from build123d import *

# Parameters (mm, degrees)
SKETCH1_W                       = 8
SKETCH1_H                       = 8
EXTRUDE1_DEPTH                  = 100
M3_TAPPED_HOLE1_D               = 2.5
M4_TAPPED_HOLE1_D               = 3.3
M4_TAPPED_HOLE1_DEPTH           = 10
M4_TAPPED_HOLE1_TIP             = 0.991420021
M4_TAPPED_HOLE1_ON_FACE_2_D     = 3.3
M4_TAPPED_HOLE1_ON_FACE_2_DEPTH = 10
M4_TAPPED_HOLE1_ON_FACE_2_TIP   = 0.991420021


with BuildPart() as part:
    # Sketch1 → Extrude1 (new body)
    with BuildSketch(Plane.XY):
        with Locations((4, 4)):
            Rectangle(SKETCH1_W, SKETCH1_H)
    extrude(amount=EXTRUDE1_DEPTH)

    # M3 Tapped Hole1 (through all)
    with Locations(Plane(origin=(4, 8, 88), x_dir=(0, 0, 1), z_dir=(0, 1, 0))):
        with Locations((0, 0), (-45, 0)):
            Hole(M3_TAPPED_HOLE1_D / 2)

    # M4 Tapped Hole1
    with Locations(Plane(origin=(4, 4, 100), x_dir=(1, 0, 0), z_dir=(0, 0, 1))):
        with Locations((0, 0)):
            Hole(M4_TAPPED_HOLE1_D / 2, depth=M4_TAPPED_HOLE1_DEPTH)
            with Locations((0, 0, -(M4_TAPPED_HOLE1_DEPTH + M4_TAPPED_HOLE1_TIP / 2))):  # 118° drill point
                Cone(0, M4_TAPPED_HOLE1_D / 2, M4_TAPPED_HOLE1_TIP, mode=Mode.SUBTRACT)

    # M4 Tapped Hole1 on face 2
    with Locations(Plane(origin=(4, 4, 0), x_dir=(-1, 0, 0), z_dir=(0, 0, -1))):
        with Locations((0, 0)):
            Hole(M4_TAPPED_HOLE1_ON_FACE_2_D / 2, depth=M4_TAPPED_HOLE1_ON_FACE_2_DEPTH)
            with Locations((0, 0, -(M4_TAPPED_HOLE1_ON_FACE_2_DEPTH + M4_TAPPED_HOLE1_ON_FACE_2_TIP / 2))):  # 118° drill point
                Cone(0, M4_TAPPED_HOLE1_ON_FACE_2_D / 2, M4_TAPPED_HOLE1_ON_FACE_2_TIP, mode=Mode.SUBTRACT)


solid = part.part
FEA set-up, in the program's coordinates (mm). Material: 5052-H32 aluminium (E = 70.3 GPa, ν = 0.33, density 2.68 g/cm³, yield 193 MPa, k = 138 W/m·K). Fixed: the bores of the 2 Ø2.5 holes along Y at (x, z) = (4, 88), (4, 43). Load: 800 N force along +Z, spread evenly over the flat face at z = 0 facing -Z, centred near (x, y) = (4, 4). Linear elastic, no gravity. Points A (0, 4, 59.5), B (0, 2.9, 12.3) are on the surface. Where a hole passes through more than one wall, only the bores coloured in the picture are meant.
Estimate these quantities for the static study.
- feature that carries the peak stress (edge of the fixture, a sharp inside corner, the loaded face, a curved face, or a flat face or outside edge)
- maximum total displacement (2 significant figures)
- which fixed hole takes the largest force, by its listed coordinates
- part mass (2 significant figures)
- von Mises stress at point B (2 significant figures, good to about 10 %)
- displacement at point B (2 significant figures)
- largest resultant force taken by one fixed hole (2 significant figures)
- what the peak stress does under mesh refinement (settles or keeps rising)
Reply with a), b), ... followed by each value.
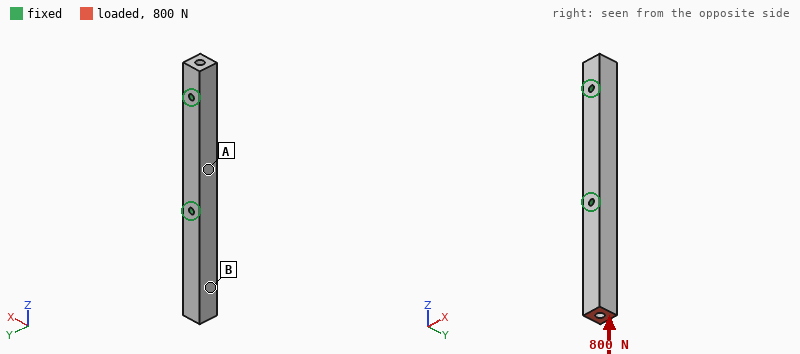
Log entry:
a) edge of the fixture
b) 8.1 µm
c) (4, 43)
d) 16 g
e) 13 MPa
f) 5.6 µm
g) 780 N
h) keeps rising
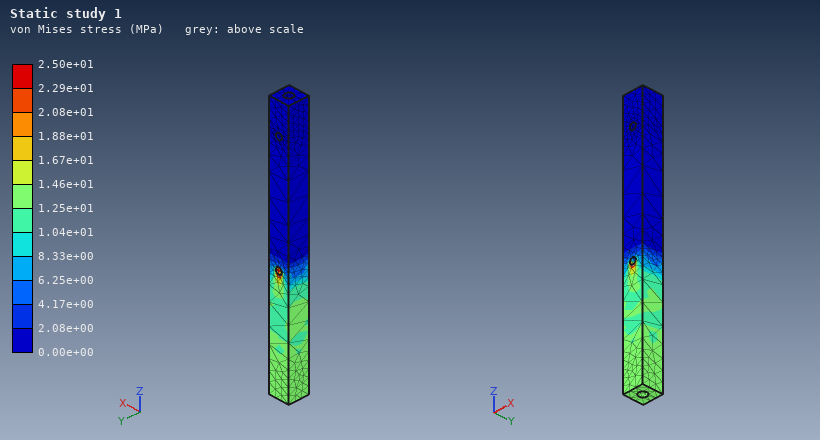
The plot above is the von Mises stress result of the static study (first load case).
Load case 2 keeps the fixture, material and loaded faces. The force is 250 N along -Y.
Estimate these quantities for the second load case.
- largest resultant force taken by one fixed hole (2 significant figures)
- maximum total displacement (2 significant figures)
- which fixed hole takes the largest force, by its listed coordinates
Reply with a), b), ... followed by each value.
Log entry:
a) 270 N
b) 0.29 mm
c) (4, 43)
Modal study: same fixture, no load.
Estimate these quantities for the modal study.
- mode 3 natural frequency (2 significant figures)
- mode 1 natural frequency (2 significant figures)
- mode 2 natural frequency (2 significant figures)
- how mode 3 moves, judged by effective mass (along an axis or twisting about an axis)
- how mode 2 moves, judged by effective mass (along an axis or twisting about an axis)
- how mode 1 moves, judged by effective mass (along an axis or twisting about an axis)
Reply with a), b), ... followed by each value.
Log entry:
a) 14 kHz
b) 3200 Hz
c) 3600 Hz
d) along X
e) along Y
f) along X
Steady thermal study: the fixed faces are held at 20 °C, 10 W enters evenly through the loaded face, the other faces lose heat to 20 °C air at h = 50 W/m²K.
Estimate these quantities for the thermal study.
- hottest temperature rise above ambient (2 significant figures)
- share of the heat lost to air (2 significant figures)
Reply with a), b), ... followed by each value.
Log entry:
a) 45 K
b) 17 %
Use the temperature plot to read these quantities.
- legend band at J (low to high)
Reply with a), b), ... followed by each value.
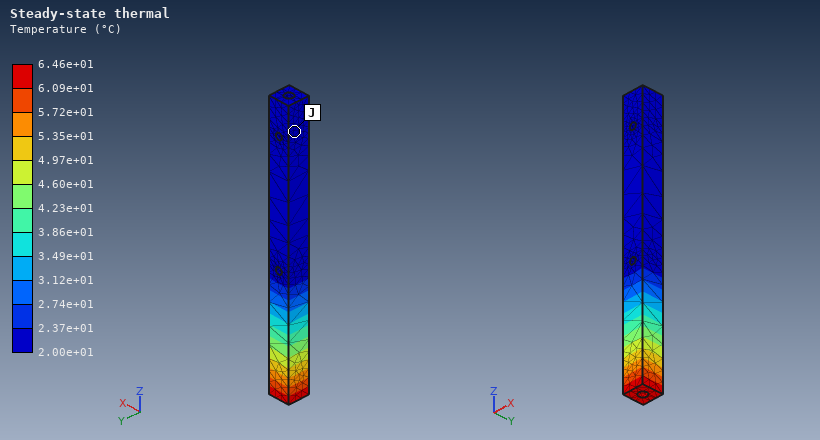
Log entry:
a) 2.00e+01 to 2.37e+01 °C
